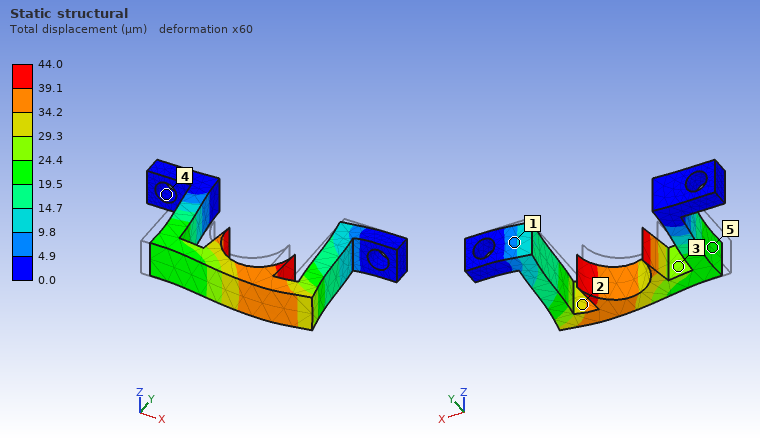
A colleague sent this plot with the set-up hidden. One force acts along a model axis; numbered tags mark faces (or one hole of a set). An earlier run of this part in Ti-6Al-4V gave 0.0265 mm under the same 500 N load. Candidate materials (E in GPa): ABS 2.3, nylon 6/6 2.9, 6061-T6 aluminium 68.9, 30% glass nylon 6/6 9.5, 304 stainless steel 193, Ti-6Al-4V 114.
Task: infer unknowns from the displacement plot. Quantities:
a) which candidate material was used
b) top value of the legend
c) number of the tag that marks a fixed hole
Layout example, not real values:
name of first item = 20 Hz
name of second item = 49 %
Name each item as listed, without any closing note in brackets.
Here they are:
which candidate material was used = 6061-T6 aluminium
top value of the legend = 44.0 µm
number of the tag that marks a fixed hole = 4
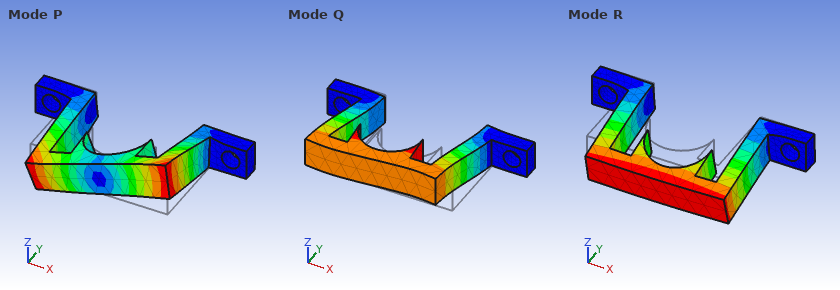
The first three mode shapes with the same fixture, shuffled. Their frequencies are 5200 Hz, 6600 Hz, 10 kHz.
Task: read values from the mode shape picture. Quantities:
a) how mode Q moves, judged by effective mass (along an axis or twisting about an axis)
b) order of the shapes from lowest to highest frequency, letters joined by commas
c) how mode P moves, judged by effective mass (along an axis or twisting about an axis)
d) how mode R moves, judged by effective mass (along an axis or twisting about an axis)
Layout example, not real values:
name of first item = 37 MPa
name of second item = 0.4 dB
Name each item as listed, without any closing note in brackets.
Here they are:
how mode Q moves, judged by effective mass = along X
order of the shapes from lowest to highest frequency, letters joined by commas = R, Q, P
how mode P moves, judged by effective mass = twisting about Y
how mode R moves, judged by effective mass = along Z
